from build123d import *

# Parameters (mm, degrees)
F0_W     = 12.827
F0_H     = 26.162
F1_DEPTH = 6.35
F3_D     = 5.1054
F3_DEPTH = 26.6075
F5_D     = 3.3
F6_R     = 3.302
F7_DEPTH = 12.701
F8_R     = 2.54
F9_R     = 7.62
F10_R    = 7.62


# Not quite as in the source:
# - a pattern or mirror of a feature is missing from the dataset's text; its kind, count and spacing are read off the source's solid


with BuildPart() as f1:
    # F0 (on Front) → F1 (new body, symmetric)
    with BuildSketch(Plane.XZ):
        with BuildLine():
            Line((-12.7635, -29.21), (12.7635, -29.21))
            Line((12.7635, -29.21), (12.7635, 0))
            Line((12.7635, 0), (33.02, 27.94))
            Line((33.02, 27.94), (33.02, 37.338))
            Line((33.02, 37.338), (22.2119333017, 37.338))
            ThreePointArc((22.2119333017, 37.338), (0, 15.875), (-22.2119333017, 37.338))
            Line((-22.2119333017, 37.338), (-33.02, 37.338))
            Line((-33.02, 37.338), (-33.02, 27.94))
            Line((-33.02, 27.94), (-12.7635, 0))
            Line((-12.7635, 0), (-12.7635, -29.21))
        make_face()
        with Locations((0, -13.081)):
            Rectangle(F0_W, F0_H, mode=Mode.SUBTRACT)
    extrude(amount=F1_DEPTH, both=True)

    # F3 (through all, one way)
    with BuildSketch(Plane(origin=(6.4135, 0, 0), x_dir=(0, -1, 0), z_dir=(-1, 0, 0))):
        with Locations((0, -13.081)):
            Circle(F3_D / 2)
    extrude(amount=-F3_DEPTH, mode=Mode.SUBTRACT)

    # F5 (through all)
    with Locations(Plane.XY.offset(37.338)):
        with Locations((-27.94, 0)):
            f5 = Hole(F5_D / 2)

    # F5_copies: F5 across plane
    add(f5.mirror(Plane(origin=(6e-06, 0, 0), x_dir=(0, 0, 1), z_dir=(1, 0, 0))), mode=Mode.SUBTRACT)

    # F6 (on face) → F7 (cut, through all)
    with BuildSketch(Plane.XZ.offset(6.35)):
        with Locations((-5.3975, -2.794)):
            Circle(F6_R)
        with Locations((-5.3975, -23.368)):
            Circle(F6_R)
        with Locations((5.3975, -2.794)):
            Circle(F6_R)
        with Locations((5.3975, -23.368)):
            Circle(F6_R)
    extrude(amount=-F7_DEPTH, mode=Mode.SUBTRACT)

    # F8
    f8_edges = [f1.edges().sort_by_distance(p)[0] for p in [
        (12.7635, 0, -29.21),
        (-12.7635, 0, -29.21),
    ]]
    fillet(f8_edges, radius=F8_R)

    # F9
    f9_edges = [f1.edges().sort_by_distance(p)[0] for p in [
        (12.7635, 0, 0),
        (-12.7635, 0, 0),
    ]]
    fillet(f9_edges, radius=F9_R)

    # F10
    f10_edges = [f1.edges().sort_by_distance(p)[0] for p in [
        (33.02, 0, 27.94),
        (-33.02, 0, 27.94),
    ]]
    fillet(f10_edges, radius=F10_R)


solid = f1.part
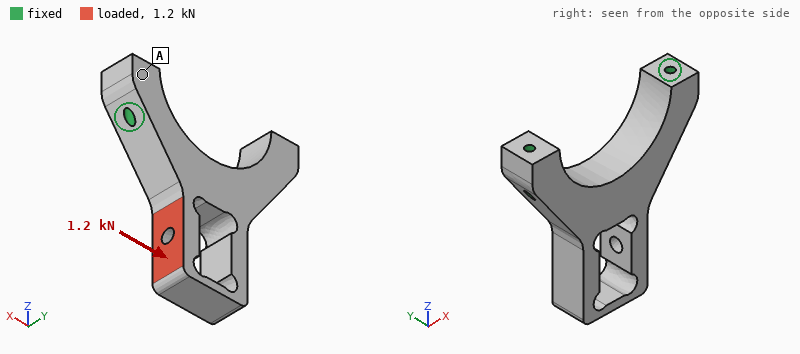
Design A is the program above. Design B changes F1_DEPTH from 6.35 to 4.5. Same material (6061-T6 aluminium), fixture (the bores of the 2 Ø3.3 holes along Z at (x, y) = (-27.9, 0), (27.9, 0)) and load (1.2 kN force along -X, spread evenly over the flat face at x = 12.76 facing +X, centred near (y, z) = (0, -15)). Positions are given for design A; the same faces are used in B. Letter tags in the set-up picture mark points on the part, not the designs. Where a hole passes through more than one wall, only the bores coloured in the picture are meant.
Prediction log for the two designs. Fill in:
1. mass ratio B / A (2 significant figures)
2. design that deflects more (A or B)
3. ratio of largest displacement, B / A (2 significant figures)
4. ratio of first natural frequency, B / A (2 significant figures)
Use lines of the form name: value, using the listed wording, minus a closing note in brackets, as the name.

mass ratio B / A: 0.70
design that deflects more: B
ratio of largest displacement, B / A: 1.4
ratio of first natural frequency, B / A: 0.80
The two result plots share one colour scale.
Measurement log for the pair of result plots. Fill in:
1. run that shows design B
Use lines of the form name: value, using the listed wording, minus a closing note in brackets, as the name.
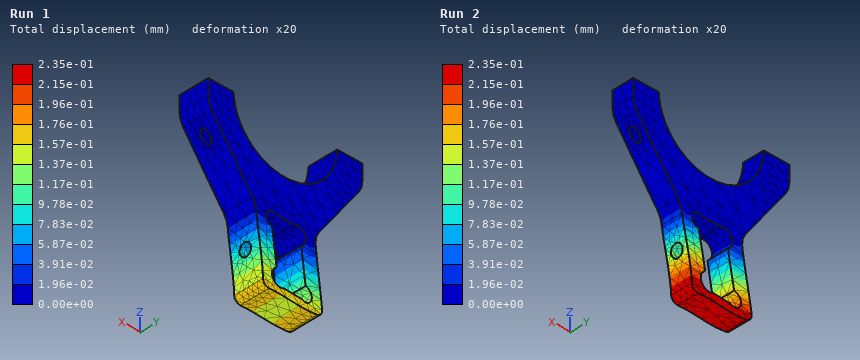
run that shows design B: Run 2
